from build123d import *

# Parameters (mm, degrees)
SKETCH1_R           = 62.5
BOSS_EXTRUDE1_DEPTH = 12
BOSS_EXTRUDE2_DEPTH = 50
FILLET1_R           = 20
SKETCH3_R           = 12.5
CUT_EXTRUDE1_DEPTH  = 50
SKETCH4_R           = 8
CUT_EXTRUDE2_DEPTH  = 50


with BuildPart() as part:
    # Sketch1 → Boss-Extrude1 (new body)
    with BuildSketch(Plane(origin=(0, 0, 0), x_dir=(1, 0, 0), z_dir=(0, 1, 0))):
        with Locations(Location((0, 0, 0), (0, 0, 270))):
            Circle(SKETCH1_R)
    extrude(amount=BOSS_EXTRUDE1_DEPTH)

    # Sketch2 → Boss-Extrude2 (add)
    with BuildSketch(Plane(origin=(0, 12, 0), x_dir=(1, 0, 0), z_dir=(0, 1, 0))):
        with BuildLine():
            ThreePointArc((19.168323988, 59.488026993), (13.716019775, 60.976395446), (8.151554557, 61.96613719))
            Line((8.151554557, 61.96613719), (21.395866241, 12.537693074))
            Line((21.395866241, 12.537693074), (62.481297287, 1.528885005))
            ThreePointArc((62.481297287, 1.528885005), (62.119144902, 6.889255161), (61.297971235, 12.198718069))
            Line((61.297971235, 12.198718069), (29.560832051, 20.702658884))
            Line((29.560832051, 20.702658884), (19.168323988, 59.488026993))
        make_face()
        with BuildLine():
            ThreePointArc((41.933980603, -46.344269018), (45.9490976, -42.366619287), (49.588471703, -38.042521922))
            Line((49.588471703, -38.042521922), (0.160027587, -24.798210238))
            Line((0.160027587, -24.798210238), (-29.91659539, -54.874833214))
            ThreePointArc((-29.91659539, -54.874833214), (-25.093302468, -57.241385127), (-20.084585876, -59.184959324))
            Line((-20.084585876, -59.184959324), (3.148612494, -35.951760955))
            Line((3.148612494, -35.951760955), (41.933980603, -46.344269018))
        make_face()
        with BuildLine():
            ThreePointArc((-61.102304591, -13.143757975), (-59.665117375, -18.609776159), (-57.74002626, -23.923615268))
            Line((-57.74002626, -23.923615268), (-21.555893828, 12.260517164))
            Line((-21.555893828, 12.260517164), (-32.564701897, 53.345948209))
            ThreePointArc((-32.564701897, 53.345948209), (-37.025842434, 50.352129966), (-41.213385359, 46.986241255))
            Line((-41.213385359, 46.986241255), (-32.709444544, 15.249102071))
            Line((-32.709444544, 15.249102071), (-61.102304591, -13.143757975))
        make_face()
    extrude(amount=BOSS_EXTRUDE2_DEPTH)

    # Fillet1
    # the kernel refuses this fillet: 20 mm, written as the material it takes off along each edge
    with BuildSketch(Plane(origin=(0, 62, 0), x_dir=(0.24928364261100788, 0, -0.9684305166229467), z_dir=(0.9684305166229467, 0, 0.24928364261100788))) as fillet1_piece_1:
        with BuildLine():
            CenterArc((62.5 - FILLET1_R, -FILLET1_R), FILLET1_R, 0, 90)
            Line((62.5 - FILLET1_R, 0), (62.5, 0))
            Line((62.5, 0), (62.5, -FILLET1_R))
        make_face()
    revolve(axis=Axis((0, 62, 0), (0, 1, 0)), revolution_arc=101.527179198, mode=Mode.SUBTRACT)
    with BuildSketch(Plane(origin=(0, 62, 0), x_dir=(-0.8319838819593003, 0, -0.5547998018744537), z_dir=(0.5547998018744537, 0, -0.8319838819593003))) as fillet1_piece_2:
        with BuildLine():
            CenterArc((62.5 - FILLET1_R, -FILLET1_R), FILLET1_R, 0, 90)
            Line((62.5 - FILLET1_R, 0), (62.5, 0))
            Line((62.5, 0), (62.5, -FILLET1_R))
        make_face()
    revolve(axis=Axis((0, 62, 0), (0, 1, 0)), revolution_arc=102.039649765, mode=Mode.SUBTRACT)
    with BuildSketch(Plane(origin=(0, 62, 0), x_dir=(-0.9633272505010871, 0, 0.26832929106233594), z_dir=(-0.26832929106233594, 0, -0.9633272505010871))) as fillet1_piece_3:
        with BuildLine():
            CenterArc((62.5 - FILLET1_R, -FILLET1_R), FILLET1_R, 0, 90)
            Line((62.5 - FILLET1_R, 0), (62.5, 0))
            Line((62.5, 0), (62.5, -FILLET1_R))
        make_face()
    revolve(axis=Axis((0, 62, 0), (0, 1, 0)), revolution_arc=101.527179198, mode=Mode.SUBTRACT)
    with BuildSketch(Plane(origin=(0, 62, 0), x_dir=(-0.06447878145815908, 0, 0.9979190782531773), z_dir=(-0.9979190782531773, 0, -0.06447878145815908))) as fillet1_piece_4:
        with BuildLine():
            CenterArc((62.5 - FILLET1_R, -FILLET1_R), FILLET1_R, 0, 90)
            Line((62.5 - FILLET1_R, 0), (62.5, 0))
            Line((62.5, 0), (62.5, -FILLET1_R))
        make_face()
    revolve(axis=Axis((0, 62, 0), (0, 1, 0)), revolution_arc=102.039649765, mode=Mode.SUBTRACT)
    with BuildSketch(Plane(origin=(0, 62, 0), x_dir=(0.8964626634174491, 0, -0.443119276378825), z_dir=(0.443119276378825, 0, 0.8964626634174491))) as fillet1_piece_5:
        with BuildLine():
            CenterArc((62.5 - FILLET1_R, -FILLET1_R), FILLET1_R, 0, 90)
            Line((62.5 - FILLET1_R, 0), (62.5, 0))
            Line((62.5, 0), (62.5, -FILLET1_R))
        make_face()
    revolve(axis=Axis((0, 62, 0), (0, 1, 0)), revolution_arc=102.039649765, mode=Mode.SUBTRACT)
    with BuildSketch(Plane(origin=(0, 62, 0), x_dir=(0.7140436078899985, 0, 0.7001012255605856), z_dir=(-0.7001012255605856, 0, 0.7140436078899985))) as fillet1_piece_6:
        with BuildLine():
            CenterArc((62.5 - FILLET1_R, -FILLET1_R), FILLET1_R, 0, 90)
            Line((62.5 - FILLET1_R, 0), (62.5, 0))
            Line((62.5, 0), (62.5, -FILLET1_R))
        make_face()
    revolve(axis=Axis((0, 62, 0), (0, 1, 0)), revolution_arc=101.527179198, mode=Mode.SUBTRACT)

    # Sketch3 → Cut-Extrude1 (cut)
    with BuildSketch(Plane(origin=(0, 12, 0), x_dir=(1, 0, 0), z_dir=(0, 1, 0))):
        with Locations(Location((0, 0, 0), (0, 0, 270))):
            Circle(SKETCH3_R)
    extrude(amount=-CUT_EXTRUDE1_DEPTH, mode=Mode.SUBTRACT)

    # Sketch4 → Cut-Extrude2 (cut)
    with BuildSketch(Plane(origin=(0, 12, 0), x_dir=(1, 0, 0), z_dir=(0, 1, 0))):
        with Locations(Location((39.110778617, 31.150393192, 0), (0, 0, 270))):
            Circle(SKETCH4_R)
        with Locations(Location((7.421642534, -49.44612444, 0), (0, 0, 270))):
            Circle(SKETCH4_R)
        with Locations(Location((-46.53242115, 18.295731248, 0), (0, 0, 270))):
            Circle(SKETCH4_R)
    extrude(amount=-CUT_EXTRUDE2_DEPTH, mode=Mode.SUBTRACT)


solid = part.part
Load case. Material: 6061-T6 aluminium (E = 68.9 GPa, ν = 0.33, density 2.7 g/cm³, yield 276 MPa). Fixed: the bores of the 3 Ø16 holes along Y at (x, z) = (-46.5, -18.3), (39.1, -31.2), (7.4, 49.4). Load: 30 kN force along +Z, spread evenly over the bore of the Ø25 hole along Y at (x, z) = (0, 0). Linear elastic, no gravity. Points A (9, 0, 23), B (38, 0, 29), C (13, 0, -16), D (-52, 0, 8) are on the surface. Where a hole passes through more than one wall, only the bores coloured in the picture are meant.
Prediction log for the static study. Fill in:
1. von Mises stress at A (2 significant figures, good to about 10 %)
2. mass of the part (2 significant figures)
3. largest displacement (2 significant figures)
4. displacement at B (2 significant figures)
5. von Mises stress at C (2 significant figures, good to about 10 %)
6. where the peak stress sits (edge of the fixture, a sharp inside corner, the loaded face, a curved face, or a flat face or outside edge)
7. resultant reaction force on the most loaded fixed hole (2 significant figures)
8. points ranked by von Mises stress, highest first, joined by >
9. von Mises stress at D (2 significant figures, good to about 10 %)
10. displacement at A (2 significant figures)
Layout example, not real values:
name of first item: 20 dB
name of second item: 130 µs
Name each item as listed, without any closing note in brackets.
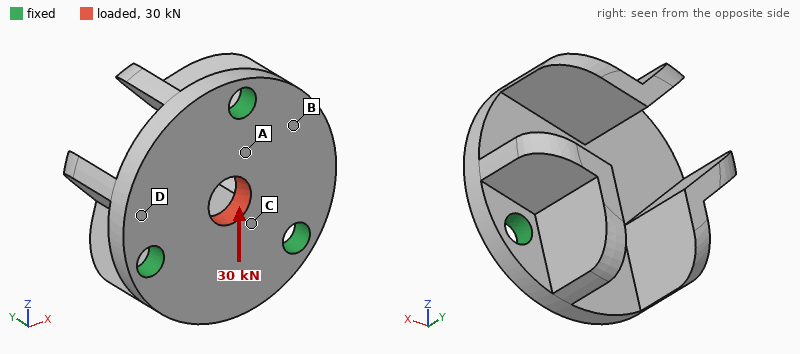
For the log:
von Mises stress at A: 33 MPa
mass of the part: 690 g
largest displacement: 23 µm
displacement at B: 6.8 µm
von Mises stress at C: 26 MPa
where the peak stress sits: edge of the fixture
resultant reaction force on the most loaded fixed hole: 11 kN
points ranked by von Mises stress, highest first, joined by >: A > C > D > B
von Mises stress at D: 11 MPa
displacement at A: 8.5 µm
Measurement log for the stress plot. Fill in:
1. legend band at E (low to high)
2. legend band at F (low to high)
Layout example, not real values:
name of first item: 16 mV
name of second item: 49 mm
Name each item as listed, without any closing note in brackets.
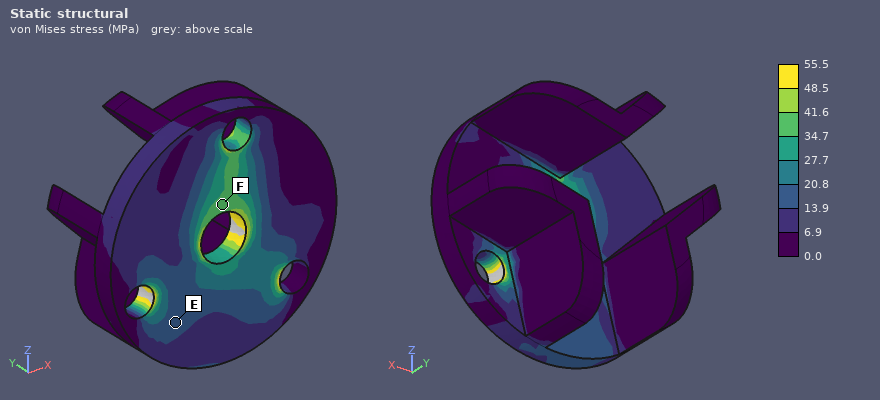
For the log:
legend band at E: 13.9 to 20.8 MPa
legend band at F: 34.7 to 41.6 MPa
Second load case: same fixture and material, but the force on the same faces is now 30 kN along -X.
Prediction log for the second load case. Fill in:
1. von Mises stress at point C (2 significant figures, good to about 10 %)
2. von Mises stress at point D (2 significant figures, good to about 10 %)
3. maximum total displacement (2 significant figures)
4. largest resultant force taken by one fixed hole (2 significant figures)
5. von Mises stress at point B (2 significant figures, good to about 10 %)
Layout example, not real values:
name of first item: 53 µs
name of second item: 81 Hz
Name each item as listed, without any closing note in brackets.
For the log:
von Mises stress at point C: 28 MPa
von Mises stress at point D: 9.8 MPa
maximum total displacement: 23 µm
largest resultant force taken by one fixed hole: 11 kN
von Mises stress at point B: 13 MPa
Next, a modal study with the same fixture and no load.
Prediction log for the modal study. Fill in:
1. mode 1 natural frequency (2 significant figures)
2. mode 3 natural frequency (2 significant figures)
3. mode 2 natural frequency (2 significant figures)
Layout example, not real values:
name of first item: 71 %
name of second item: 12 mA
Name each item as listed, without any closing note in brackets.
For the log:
mode 1 natural frequency: 3200 Hz
mode 3 natural frequency: 3700 Hz
mode 2 natural frequency: 3700 Hz
